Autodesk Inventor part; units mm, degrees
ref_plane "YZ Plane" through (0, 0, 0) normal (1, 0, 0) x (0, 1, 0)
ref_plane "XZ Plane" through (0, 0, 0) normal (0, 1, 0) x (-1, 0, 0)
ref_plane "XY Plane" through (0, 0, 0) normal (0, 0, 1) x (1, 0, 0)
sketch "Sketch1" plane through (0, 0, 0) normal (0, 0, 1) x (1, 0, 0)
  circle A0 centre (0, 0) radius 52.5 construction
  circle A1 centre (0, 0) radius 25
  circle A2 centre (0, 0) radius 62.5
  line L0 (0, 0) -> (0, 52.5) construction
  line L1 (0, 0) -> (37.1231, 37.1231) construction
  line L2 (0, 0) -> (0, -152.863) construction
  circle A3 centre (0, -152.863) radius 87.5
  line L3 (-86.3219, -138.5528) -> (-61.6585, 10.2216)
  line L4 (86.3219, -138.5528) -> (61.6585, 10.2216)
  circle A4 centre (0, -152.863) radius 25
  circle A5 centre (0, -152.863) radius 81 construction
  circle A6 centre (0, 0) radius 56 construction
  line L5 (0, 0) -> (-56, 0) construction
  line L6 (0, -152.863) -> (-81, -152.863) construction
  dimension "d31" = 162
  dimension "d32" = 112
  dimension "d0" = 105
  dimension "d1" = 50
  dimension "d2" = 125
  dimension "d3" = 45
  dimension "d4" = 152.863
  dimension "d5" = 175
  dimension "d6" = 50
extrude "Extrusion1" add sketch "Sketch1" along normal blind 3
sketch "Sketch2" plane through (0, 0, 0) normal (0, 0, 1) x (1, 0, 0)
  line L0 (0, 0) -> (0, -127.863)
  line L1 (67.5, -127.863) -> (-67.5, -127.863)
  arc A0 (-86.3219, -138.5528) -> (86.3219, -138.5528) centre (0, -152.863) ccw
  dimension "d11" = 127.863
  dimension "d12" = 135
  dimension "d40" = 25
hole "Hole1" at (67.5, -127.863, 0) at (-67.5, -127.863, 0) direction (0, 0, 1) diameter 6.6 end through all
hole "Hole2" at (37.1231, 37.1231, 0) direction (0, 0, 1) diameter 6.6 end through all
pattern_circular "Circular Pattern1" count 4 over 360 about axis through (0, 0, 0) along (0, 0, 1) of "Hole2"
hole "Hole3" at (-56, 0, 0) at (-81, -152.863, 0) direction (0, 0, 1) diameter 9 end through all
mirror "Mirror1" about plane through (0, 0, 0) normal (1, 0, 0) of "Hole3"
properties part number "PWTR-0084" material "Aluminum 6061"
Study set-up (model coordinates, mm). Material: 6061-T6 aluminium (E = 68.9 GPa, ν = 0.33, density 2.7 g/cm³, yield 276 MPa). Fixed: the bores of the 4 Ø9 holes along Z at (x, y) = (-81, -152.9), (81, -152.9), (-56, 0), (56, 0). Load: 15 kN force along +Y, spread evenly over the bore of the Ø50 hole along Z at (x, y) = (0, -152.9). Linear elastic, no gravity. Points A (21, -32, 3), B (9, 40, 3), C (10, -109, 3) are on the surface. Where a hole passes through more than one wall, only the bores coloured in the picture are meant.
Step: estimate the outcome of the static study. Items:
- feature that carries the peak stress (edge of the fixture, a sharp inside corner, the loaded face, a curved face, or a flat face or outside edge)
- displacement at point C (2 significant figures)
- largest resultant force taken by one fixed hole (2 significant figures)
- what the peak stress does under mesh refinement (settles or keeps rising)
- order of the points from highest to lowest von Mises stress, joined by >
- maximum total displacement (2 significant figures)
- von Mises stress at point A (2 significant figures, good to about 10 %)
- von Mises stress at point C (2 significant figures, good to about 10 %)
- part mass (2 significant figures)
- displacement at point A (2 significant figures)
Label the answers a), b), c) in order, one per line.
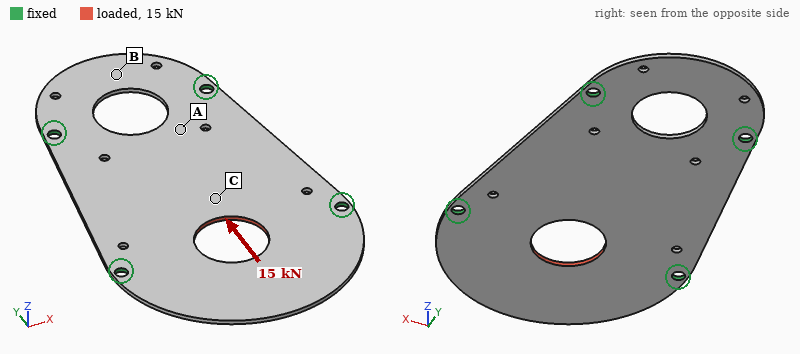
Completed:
a) edge of the fixture
b) 40 µm
c) 4.7 kN
d) keeps rising
e) C > A > B
f) 69 µm
g) 15 MPa
h) 33 MPa
i) 300 g
j) 18 µm
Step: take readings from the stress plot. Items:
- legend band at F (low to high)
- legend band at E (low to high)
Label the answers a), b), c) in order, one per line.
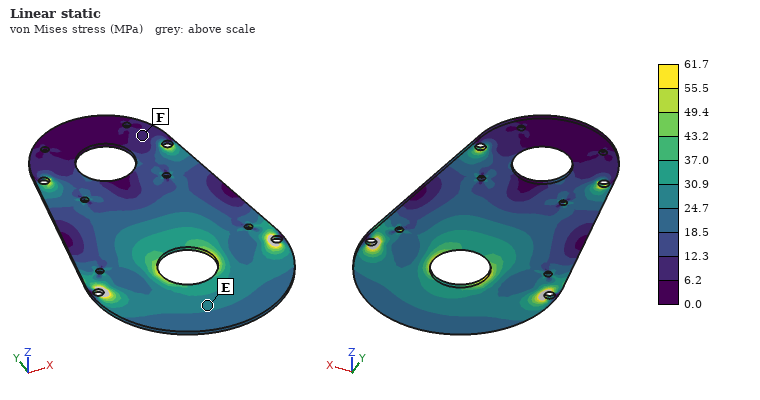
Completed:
a) 6.2 to 12.3 MPa
b) 24.7 to 30.9 MPa
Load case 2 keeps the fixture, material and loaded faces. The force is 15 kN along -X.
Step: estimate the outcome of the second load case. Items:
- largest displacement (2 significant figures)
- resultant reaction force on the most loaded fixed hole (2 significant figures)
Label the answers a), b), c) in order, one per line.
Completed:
a) 61 µm
b) 6.7 kN
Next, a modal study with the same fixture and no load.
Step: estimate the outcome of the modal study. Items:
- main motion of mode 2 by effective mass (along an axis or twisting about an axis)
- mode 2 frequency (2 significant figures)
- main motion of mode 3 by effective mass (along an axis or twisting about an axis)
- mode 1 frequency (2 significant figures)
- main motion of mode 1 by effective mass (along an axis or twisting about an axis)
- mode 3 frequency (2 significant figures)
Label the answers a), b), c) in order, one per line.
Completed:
a) along Z
b) 480 Hz
c) along Z
d) 280 Hz
e) along Z
f) 580 Hz
